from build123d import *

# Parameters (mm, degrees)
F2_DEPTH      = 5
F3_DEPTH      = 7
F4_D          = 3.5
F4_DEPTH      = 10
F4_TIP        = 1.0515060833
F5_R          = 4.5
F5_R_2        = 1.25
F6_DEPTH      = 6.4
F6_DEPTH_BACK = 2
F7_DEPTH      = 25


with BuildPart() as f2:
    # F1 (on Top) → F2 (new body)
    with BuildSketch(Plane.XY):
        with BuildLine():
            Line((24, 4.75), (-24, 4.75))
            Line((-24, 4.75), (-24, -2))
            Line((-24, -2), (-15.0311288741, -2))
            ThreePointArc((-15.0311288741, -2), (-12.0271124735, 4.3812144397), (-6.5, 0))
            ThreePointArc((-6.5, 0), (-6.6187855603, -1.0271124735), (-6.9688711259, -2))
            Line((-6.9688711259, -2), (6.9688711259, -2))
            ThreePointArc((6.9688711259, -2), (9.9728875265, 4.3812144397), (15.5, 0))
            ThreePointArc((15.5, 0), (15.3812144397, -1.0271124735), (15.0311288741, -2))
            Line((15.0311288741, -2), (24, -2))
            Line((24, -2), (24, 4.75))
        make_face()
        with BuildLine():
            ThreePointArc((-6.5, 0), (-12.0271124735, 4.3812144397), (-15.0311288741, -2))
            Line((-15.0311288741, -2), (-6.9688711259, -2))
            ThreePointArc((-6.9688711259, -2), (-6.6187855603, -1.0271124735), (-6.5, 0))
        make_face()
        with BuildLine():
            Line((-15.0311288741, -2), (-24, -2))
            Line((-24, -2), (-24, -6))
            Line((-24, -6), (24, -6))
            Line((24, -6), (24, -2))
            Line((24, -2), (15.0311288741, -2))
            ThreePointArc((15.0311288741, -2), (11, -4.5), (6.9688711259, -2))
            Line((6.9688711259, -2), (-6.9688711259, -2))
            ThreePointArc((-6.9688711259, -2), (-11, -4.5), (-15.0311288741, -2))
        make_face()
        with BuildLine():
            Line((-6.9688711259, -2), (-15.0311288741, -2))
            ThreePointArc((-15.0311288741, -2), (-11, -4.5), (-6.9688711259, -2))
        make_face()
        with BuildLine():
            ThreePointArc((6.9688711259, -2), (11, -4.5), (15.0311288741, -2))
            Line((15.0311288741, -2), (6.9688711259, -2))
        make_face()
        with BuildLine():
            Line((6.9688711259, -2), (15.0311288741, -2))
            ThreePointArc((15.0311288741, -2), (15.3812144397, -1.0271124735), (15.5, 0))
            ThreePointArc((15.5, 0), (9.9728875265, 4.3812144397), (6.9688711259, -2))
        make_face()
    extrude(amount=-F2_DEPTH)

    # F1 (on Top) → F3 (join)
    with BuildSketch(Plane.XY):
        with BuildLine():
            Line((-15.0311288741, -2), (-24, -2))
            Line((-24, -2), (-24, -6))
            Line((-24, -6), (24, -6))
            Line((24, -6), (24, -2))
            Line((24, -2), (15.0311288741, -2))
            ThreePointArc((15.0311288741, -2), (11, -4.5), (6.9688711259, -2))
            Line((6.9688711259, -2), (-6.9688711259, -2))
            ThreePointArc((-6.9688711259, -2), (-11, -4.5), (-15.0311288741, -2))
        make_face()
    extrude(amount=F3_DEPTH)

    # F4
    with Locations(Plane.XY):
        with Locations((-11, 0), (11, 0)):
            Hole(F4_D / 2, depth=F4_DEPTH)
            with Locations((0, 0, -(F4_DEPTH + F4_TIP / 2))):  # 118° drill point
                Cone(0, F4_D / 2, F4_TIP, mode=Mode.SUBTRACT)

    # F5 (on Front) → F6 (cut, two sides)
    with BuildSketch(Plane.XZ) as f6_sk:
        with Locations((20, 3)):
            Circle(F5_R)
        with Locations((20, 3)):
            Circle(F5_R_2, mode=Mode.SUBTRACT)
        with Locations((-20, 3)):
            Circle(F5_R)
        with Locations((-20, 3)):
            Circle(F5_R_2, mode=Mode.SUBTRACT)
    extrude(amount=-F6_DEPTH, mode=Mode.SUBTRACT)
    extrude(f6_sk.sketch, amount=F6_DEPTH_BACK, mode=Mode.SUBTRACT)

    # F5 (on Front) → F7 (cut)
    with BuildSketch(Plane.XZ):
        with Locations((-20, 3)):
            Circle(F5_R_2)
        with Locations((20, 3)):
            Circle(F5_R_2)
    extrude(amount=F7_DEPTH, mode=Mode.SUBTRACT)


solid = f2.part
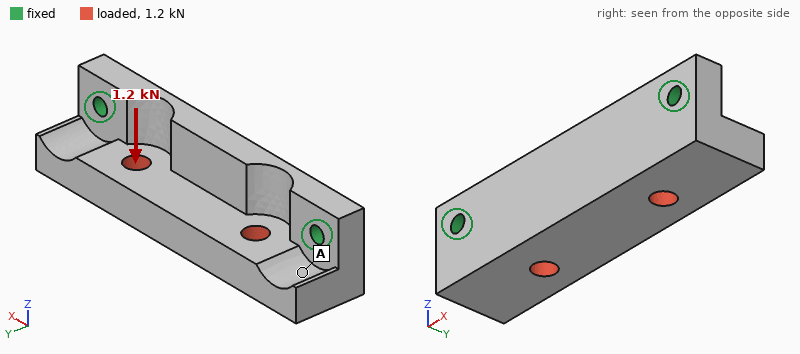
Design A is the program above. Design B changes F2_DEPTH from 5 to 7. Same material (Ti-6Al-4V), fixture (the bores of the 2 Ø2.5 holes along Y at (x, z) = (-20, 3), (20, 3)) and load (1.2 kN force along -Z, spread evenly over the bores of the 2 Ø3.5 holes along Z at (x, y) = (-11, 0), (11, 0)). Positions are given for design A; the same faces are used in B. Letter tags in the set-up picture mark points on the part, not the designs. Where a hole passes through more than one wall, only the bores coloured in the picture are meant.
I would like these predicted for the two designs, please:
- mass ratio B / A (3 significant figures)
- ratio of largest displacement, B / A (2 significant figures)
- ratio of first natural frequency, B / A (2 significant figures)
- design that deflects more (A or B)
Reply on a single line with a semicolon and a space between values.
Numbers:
1.28; 0.84; 0.83; A
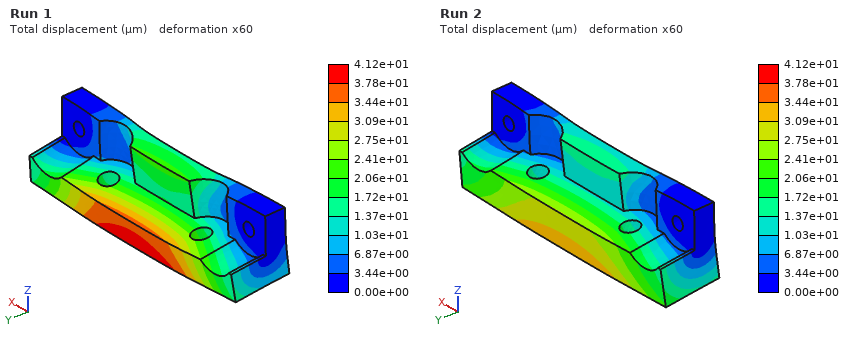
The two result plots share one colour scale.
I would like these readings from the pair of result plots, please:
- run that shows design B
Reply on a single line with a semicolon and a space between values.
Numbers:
Run 2
